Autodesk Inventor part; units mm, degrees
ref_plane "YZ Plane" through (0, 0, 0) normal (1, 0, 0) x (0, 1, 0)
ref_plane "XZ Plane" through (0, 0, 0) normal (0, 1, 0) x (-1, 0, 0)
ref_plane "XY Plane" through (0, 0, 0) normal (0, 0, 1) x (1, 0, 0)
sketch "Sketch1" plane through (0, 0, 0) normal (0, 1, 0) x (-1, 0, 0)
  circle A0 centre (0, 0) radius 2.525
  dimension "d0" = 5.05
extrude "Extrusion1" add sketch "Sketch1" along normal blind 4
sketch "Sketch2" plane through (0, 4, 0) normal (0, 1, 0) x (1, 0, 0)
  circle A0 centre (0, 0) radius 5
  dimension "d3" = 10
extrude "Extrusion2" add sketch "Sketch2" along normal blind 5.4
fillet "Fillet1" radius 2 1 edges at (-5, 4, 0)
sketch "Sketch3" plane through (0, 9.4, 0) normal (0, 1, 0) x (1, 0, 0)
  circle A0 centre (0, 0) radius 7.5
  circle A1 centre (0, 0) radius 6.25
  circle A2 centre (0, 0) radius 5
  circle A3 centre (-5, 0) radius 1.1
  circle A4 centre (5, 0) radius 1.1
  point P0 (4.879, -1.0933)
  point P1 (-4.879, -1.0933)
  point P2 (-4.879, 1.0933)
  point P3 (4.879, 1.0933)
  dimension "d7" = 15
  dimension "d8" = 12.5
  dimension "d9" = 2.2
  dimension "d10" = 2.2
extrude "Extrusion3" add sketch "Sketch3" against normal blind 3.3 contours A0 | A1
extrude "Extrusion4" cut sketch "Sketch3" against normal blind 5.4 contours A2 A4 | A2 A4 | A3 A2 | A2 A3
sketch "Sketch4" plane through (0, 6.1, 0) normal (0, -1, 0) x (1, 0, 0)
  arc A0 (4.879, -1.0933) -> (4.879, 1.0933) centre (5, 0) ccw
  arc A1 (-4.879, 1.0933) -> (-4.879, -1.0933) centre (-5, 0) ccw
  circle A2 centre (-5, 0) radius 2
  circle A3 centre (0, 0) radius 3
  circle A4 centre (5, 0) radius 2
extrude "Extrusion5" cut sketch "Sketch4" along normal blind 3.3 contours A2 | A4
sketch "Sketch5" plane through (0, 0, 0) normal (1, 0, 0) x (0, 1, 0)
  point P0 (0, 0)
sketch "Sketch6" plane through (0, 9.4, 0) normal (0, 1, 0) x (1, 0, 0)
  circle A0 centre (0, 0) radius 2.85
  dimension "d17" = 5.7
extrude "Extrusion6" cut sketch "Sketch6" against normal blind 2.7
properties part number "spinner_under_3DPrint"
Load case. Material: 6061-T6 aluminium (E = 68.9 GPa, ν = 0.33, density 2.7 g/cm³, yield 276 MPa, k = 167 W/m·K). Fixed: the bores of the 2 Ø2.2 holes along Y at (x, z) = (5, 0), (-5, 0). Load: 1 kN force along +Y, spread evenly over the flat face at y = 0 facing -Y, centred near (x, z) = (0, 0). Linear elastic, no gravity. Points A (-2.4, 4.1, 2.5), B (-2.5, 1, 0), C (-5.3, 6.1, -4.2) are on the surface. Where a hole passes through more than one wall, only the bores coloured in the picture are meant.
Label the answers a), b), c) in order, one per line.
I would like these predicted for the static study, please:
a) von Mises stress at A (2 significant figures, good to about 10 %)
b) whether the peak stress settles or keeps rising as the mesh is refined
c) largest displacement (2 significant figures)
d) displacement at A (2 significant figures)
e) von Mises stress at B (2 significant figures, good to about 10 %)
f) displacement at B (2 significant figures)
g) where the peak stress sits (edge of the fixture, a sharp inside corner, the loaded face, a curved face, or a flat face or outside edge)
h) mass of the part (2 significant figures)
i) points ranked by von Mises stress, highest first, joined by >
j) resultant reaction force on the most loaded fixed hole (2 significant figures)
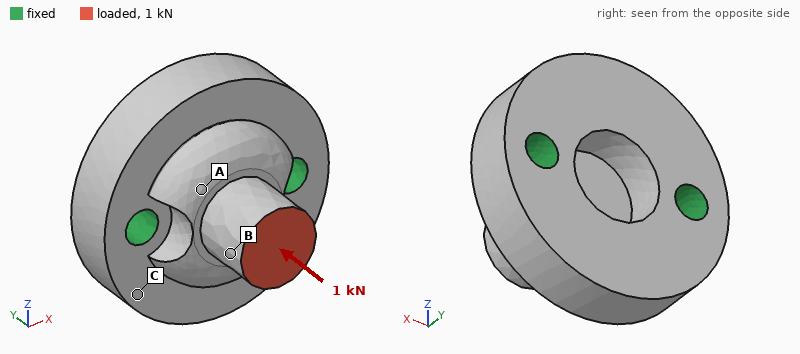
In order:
a) 23 MPa
b) keeps rising
c) 7.7 µm
d) 3.2 µm
e) 49 MPa
f) 7.0 µm
g) edge of the fixture
h) 1.9 g
i) B > A > C
j) 530 N
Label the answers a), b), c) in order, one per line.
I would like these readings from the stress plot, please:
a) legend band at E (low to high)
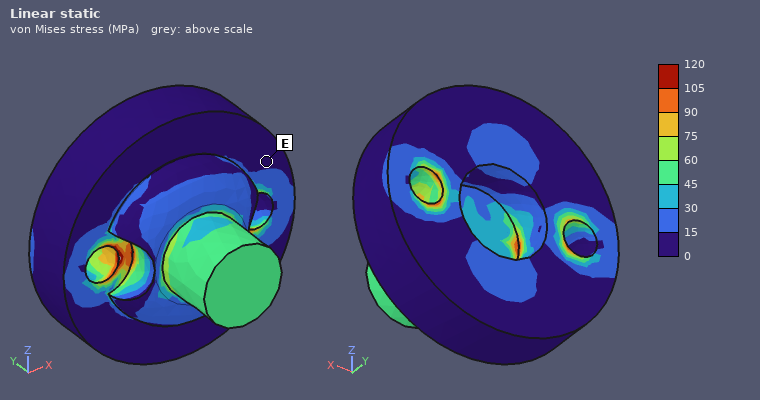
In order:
a) 0 to 15 MPa
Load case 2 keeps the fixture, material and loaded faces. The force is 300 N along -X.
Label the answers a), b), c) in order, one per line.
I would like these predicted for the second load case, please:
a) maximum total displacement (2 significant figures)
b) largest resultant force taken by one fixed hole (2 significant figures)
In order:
a) 13 µm
b) 290 N
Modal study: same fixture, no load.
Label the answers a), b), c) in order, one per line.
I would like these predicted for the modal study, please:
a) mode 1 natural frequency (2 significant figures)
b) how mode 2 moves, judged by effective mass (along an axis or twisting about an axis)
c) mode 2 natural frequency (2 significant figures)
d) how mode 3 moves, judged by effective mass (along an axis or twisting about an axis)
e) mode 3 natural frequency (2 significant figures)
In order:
a) 39 kHz
b) along Y
c) 61 kHz
d) along X
e) 76 kHz
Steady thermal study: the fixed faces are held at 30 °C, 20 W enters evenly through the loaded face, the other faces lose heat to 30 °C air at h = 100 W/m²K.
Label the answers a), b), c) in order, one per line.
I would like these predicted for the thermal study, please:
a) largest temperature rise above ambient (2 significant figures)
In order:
a) 40 K
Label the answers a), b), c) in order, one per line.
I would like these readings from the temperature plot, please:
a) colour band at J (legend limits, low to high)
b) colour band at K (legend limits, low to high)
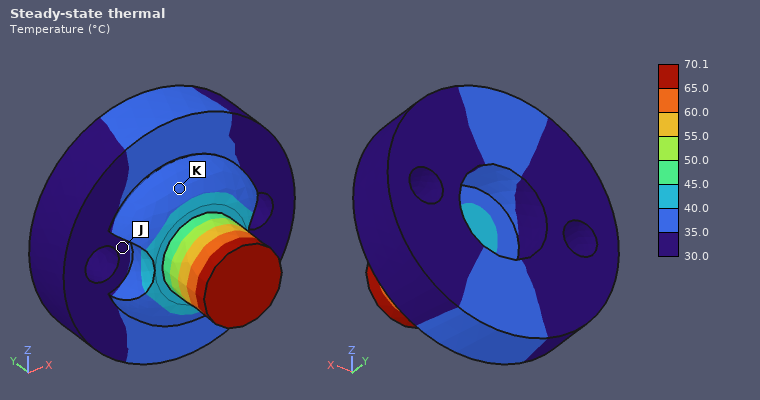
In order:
a) 30.0 to 35.0 °C
b) 35.0 to 40.0 °C
